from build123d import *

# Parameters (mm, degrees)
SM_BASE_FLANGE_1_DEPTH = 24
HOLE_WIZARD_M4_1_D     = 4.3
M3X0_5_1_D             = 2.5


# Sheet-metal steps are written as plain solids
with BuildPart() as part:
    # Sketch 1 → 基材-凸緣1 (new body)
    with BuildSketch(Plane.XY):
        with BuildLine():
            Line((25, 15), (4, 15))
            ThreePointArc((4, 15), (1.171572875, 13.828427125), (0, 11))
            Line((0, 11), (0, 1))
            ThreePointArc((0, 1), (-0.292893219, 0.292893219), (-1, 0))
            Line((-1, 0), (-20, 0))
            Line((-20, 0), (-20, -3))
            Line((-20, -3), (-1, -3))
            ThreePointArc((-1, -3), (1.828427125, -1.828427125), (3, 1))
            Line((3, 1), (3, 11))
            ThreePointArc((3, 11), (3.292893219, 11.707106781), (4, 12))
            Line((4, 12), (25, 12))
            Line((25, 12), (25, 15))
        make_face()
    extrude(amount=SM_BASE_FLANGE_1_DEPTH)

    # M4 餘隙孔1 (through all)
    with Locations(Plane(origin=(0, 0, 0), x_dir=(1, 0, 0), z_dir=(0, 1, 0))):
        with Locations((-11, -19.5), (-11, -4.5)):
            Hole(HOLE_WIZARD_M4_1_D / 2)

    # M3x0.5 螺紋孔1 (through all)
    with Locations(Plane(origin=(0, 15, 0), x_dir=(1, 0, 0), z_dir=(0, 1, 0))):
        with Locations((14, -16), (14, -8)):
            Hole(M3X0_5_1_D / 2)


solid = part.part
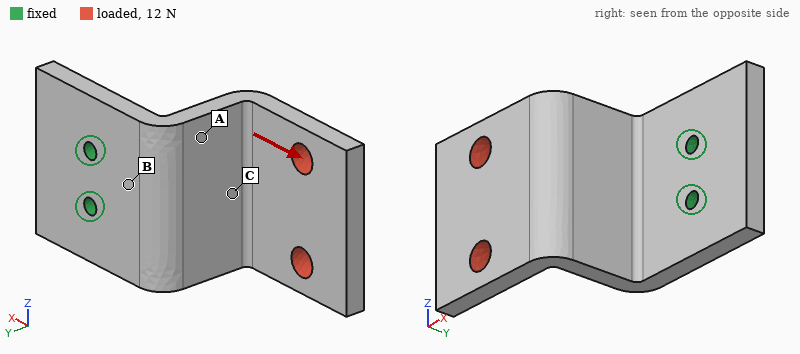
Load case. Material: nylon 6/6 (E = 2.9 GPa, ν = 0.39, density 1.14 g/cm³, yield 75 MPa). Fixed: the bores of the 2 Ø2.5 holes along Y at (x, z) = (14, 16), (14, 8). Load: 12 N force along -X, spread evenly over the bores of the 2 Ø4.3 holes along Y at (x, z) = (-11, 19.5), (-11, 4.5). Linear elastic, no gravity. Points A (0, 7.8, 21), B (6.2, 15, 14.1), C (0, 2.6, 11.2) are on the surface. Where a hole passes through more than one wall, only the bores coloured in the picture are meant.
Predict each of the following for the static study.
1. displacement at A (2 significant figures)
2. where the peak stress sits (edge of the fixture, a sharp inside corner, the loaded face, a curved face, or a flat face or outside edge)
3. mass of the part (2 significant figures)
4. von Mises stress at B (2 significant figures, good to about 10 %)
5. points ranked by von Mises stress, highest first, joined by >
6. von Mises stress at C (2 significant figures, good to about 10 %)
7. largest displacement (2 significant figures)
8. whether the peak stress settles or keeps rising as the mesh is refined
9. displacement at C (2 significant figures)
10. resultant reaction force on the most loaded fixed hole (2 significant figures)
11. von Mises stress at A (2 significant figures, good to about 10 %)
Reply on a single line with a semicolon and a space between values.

0.14 mm; edge of the fixture; 4.6 g; 4.4 MPa; B > A > C; 1.2 MPa; 0.60 mm; keeps rising; 0.21 mm; 6.3 N; 2.9 MPa
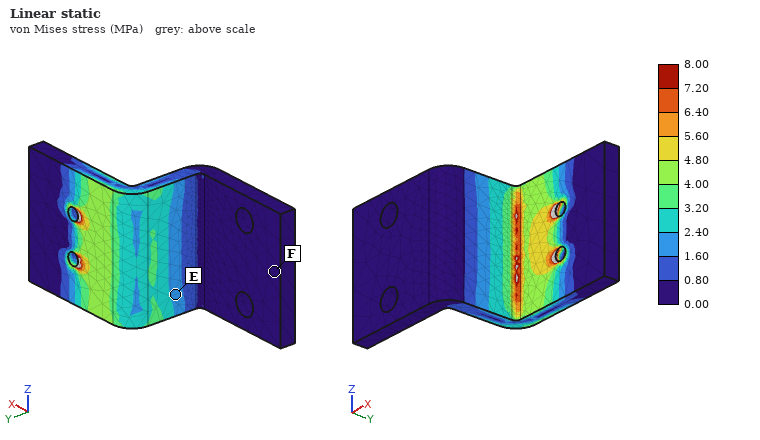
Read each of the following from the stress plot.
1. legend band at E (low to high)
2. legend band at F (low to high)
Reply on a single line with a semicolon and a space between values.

1.60 to 2.40 MPa; 0.00 to 0.80 MPa
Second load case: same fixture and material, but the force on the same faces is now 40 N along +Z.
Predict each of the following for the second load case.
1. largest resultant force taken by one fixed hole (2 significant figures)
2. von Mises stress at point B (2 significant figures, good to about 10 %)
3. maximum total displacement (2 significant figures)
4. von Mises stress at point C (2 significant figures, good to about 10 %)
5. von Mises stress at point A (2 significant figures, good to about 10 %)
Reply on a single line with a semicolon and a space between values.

110 N; 3.8 MPa; 0.63 mm; 8.3 MPa; 7.2 MPa
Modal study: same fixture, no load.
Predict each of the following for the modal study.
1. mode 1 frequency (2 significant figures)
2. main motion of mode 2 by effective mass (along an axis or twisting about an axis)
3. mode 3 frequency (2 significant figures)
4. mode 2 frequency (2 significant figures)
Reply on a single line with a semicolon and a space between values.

480 Hz; along Z; 1500 Hz; 1100 Hz
